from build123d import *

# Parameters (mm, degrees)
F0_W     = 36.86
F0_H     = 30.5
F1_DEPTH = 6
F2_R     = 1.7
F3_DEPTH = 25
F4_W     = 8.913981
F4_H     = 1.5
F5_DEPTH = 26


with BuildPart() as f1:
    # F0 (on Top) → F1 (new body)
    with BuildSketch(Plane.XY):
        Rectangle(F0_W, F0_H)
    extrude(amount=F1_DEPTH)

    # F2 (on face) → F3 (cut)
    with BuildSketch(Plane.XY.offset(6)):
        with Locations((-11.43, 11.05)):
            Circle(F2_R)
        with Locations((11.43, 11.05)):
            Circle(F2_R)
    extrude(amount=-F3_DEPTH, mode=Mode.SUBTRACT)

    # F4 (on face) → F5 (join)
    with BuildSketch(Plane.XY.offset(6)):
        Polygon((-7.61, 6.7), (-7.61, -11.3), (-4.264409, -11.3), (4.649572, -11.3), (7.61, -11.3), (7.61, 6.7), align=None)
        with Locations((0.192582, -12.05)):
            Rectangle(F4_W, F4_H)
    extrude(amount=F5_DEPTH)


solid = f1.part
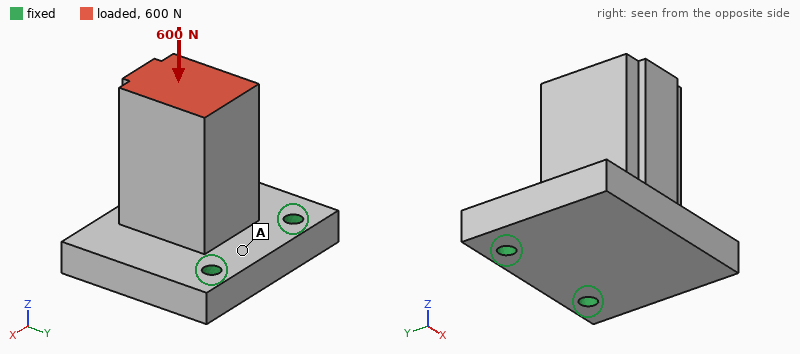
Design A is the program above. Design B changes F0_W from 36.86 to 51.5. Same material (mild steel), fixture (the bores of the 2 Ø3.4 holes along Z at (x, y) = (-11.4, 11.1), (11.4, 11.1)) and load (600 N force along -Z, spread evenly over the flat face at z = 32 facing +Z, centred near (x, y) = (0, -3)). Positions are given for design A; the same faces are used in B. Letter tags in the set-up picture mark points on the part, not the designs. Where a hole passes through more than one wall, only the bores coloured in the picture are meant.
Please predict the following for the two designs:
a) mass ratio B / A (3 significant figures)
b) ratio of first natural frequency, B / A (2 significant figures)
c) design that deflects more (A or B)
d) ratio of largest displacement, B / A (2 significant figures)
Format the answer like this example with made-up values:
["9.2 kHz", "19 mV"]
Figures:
["1.19", "1.0", "A", "0.90"]
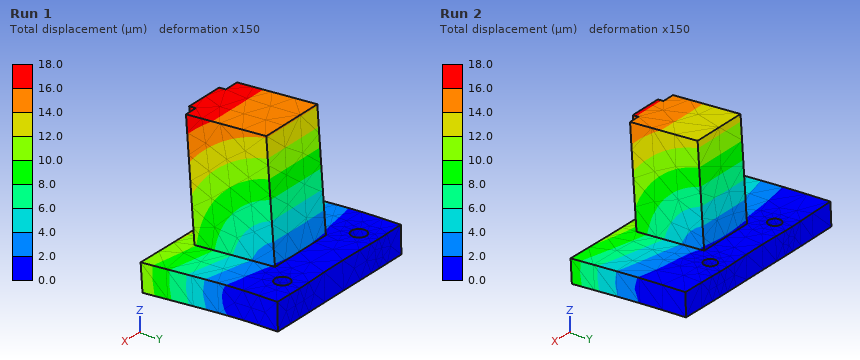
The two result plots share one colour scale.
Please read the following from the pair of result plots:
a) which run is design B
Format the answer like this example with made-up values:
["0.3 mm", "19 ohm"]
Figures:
["Run 2"]
